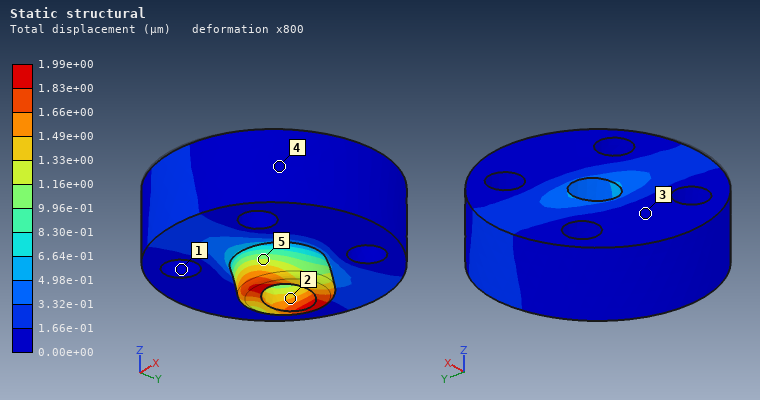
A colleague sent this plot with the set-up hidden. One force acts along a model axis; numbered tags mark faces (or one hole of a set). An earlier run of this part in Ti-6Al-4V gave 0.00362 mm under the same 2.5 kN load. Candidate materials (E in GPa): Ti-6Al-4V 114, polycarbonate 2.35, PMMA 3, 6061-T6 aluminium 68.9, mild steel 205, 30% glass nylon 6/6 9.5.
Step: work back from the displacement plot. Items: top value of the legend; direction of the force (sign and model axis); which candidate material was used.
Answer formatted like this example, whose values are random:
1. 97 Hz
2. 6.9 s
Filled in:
1. 1.99e+00 µm
2. +Y
3. mild steel
